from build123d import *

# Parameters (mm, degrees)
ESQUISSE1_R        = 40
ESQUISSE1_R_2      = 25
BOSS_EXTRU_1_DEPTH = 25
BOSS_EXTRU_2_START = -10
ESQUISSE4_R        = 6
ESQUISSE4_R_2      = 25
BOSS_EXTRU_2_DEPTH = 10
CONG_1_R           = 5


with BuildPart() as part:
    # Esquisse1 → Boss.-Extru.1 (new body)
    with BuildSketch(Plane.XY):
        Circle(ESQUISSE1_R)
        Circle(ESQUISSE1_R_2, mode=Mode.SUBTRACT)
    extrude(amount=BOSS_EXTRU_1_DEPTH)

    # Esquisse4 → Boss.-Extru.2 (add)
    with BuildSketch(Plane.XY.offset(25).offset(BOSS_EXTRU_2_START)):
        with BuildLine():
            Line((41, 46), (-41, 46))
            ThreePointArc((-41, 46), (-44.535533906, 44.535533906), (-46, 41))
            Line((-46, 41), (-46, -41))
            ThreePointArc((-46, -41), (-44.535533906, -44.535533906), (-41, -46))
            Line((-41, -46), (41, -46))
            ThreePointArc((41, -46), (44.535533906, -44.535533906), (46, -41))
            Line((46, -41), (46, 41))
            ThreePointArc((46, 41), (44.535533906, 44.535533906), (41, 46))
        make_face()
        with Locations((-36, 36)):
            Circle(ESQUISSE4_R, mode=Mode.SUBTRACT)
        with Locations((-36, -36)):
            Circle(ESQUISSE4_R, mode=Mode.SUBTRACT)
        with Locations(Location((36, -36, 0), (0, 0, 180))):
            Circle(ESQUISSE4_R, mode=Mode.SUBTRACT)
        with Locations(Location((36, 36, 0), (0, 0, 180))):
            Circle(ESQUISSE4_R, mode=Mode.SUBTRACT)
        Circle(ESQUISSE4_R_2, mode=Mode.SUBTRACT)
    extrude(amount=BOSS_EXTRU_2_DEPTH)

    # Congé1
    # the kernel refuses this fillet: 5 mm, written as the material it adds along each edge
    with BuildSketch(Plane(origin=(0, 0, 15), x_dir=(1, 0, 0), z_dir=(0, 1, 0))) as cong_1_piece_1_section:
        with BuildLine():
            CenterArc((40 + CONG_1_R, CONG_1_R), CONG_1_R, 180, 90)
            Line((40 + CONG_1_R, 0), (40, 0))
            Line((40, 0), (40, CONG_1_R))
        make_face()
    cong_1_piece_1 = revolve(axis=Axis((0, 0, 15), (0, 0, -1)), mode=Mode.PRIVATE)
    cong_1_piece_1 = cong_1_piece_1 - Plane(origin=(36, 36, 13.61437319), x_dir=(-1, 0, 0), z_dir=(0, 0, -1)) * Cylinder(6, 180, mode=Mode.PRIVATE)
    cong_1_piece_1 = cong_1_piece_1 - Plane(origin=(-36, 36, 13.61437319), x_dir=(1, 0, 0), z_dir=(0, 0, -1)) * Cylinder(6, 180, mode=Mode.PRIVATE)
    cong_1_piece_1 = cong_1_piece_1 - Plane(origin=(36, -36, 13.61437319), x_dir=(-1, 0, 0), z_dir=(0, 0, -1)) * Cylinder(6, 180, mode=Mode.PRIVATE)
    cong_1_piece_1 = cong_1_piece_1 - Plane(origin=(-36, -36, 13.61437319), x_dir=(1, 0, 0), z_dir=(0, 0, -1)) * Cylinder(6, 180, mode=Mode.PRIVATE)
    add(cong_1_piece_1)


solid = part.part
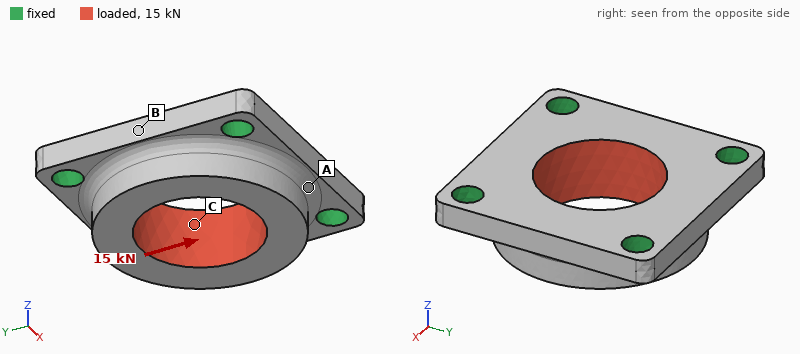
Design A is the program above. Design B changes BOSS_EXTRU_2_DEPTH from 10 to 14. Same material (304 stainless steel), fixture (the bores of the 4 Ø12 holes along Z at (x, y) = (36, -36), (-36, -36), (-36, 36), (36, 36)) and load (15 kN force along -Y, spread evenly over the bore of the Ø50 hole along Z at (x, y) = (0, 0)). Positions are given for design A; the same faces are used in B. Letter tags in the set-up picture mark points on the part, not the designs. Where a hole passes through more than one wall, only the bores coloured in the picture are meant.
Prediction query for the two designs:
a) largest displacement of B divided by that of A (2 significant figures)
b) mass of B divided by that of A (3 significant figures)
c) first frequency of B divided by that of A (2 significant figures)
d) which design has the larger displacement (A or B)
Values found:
0.80
1.22
1.1
A
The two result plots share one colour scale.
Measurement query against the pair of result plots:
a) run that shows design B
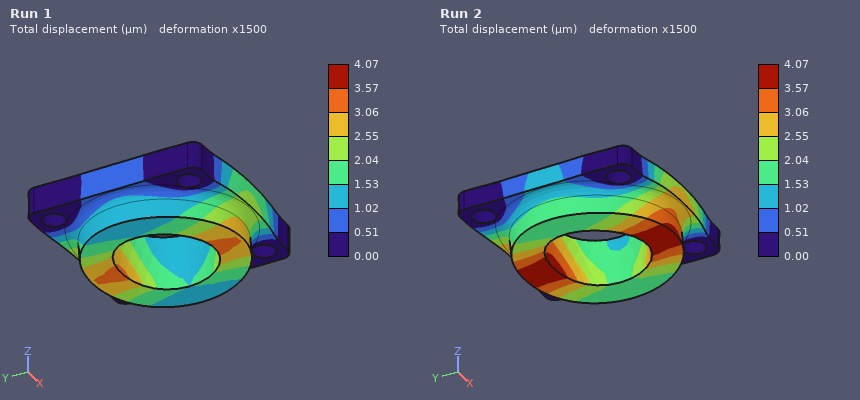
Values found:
Run 1
